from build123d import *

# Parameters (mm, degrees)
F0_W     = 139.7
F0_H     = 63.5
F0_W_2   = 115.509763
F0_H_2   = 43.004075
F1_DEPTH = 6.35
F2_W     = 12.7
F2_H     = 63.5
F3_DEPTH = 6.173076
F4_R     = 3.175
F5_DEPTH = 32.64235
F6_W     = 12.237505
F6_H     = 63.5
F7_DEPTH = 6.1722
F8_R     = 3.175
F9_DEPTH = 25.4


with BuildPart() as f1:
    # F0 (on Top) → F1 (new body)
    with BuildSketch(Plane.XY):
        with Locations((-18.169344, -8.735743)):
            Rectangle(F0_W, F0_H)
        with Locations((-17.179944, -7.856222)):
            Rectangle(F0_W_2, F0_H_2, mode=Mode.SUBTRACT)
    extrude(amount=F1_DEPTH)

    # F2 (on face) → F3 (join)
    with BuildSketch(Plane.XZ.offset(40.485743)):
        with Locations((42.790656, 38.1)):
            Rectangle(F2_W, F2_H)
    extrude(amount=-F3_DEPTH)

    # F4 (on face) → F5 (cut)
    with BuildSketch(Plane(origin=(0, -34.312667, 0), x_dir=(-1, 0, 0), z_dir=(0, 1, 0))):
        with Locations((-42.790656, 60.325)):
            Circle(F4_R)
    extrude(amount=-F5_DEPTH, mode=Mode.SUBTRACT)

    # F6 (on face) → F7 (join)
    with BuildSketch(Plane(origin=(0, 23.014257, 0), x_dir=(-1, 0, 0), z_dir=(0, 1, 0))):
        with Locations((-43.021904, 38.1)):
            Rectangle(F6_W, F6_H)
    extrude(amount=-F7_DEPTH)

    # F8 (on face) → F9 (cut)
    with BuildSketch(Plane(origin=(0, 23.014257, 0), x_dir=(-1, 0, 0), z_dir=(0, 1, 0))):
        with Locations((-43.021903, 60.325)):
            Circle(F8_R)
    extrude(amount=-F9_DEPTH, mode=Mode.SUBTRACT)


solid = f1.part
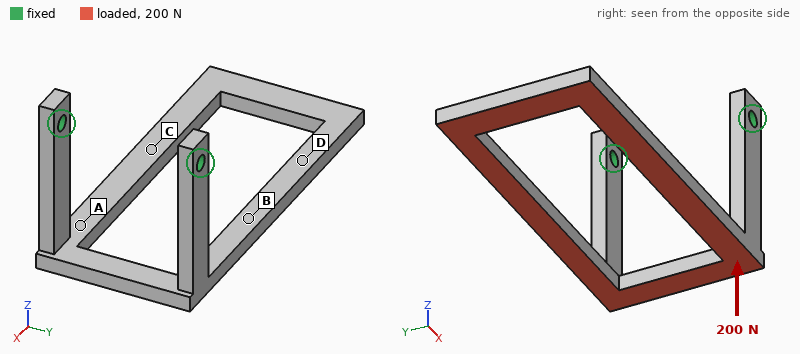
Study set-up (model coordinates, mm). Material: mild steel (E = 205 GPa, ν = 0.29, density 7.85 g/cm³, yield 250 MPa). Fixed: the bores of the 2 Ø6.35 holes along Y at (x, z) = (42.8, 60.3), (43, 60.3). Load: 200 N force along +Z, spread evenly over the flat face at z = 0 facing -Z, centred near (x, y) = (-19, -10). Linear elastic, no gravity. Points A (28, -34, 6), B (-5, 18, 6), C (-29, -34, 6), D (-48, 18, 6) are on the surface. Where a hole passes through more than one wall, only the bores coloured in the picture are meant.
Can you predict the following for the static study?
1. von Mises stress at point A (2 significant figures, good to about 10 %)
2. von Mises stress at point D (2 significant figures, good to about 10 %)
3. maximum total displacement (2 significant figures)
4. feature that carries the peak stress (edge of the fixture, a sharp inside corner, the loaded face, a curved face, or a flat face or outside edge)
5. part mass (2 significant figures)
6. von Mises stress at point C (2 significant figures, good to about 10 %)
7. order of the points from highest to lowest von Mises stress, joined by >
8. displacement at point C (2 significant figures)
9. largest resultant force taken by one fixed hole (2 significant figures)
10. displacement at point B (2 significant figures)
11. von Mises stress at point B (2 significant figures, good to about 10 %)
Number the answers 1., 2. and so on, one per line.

1. 73 MPa
2. 13 MPa
3. 0.84 mm
4. the loaded face
5. 270 g
6. 24 MPa
7. A > B > C > D
8. 0.36 mm
9. 110 N
10. 0.20 mm
11. 43 MPa
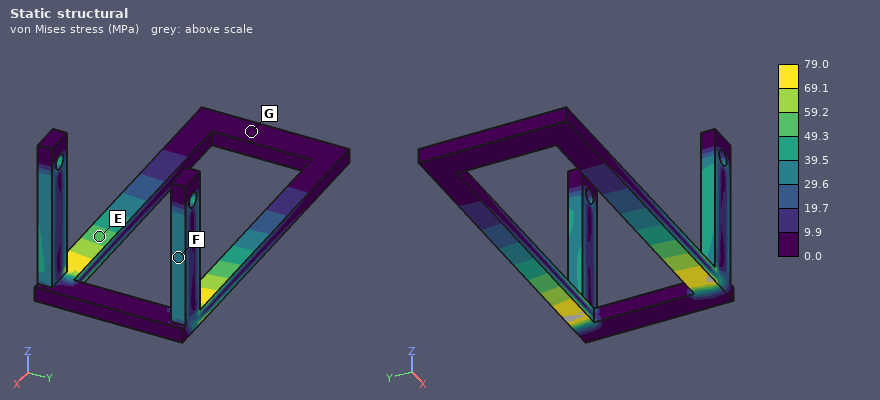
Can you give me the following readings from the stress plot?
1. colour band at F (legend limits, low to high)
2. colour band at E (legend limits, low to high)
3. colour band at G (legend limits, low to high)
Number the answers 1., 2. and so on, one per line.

1. 29.6 to 39.5 MPa
2. 49.3 to 59.2 MPa
3. 0.0 to 9.9 MPa
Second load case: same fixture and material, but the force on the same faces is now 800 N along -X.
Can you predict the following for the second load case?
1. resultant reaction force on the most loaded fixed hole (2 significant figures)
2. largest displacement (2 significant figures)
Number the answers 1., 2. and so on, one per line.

1. 420 N
2. 0.64 mm
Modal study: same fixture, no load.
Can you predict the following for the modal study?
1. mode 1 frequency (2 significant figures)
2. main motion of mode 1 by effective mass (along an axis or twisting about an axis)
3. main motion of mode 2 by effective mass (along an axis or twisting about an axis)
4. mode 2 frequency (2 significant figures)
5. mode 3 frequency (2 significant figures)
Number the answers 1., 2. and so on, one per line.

1. 200 Hz
2. along Z
3. along Y
4. 340 Hz
5. 760 Hz
